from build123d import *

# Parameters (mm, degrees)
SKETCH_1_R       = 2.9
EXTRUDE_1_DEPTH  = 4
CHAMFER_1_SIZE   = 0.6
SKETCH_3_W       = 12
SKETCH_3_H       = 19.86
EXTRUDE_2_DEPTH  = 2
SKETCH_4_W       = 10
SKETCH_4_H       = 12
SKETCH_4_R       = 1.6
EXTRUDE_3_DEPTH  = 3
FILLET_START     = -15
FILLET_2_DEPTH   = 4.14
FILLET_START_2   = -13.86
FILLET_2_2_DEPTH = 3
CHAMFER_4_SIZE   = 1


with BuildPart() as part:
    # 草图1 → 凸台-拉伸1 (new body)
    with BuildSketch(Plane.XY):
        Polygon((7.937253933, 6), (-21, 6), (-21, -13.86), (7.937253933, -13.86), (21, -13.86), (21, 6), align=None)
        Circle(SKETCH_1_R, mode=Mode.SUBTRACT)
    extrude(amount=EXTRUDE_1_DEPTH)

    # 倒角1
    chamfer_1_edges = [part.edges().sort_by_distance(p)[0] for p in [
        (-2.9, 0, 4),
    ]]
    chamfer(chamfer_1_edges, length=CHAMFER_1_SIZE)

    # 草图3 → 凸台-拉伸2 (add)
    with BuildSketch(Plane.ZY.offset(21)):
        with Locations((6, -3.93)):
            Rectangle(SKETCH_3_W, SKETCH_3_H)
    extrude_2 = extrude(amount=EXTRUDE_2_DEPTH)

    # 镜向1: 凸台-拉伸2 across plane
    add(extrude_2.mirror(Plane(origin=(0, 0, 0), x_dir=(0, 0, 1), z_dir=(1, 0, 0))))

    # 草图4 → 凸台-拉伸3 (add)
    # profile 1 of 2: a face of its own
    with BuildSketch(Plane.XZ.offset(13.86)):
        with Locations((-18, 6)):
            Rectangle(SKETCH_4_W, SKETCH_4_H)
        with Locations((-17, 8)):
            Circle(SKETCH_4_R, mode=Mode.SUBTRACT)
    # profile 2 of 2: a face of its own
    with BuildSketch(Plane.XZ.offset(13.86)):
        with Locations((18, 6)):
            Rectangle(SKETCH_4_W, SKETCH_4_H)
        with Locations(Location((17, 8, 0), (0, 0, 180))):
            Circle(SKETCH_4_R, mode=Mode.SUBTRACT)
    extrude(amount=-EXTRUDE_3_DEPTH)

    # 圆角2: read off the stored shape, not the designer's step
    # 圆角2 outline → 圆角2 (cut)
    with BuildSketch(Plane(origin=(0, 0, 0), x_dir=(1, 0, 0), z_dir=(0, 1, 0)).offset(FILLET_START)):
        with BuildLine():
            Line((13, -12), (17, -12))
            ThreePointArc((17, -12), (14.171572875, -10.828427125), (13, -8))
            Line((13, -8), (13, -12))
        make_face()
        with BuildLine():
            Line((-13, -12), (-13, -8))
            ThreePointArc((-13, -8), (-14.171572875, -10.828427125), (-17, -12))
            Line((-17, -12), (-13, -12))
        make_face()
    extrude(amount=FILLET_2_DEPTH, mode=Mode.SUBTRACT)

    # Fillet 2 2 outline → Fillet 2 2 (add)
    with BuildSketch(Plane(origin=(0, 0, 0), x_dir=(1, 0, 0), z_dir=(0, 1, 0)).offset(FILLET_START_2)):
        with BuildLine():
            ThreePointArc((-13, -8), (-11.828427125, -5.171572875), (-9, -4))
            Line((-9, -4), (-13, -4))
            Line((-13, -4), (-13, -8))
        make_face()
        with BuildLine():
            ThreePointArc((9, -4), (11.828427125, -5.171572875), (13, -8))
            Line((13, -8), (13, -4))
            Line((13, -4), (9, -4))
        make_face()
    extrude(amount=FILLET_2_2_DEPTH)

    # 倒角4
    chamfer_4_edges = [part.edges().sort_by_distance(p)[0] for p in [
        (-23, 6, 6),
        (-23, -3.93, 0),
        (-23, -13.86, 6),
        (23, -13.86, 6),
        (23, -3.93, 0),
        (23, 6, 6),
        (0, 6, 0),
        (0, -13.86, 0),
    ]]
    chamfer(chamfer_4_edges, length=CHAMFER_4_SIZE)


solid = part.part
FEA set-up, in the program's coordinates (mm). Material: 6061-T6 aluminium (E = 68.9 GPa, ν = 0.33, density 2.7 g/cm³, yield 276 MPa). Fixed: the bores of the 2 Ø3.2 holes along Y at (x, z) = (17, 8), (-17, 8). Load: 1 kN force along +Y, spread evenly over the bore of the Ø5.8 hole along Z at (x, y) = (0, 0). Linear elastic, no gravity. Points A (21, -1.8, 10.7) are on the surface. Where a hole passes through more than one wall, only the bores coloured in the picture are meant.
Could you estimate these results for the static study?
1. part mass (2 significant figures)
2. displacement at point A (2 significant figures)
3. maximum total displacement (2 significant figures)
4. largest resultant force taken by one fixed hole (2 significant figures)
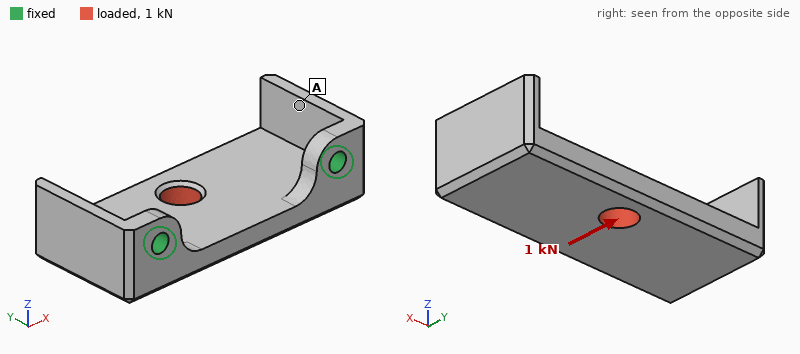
12 g
31 µm
72 µm
520 N
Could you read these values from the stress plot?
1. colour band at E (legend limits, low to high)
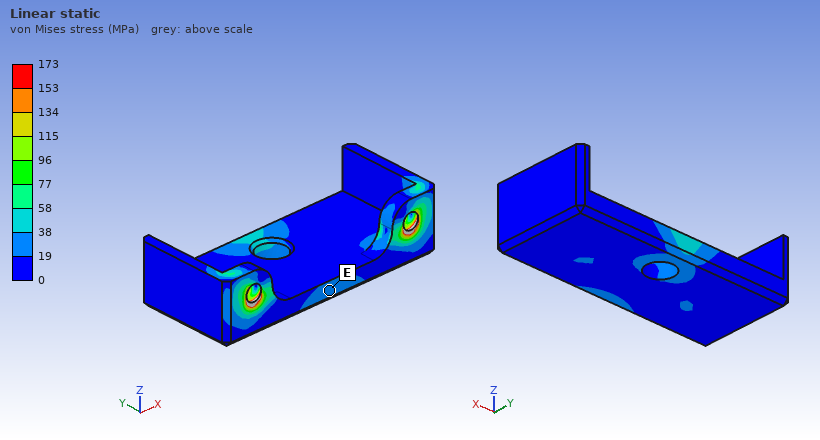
19 to 38 MPa
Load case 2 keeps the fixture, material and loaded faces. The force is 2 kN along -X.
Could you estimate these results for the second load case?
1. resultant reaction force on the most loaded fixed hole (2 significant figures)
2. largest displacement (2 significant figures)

1.2 kN
51 µm
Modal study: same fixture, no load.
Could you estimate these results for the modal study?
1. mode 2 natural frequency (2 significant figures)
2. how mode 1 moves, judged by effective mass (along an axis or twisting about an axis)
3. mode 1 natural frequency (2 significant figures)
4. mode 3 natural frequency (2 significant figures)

8400 Hz
along Z
4800 Hz
14 kHz
